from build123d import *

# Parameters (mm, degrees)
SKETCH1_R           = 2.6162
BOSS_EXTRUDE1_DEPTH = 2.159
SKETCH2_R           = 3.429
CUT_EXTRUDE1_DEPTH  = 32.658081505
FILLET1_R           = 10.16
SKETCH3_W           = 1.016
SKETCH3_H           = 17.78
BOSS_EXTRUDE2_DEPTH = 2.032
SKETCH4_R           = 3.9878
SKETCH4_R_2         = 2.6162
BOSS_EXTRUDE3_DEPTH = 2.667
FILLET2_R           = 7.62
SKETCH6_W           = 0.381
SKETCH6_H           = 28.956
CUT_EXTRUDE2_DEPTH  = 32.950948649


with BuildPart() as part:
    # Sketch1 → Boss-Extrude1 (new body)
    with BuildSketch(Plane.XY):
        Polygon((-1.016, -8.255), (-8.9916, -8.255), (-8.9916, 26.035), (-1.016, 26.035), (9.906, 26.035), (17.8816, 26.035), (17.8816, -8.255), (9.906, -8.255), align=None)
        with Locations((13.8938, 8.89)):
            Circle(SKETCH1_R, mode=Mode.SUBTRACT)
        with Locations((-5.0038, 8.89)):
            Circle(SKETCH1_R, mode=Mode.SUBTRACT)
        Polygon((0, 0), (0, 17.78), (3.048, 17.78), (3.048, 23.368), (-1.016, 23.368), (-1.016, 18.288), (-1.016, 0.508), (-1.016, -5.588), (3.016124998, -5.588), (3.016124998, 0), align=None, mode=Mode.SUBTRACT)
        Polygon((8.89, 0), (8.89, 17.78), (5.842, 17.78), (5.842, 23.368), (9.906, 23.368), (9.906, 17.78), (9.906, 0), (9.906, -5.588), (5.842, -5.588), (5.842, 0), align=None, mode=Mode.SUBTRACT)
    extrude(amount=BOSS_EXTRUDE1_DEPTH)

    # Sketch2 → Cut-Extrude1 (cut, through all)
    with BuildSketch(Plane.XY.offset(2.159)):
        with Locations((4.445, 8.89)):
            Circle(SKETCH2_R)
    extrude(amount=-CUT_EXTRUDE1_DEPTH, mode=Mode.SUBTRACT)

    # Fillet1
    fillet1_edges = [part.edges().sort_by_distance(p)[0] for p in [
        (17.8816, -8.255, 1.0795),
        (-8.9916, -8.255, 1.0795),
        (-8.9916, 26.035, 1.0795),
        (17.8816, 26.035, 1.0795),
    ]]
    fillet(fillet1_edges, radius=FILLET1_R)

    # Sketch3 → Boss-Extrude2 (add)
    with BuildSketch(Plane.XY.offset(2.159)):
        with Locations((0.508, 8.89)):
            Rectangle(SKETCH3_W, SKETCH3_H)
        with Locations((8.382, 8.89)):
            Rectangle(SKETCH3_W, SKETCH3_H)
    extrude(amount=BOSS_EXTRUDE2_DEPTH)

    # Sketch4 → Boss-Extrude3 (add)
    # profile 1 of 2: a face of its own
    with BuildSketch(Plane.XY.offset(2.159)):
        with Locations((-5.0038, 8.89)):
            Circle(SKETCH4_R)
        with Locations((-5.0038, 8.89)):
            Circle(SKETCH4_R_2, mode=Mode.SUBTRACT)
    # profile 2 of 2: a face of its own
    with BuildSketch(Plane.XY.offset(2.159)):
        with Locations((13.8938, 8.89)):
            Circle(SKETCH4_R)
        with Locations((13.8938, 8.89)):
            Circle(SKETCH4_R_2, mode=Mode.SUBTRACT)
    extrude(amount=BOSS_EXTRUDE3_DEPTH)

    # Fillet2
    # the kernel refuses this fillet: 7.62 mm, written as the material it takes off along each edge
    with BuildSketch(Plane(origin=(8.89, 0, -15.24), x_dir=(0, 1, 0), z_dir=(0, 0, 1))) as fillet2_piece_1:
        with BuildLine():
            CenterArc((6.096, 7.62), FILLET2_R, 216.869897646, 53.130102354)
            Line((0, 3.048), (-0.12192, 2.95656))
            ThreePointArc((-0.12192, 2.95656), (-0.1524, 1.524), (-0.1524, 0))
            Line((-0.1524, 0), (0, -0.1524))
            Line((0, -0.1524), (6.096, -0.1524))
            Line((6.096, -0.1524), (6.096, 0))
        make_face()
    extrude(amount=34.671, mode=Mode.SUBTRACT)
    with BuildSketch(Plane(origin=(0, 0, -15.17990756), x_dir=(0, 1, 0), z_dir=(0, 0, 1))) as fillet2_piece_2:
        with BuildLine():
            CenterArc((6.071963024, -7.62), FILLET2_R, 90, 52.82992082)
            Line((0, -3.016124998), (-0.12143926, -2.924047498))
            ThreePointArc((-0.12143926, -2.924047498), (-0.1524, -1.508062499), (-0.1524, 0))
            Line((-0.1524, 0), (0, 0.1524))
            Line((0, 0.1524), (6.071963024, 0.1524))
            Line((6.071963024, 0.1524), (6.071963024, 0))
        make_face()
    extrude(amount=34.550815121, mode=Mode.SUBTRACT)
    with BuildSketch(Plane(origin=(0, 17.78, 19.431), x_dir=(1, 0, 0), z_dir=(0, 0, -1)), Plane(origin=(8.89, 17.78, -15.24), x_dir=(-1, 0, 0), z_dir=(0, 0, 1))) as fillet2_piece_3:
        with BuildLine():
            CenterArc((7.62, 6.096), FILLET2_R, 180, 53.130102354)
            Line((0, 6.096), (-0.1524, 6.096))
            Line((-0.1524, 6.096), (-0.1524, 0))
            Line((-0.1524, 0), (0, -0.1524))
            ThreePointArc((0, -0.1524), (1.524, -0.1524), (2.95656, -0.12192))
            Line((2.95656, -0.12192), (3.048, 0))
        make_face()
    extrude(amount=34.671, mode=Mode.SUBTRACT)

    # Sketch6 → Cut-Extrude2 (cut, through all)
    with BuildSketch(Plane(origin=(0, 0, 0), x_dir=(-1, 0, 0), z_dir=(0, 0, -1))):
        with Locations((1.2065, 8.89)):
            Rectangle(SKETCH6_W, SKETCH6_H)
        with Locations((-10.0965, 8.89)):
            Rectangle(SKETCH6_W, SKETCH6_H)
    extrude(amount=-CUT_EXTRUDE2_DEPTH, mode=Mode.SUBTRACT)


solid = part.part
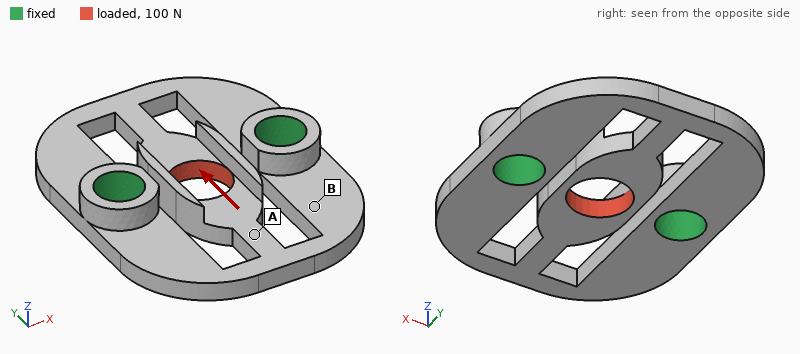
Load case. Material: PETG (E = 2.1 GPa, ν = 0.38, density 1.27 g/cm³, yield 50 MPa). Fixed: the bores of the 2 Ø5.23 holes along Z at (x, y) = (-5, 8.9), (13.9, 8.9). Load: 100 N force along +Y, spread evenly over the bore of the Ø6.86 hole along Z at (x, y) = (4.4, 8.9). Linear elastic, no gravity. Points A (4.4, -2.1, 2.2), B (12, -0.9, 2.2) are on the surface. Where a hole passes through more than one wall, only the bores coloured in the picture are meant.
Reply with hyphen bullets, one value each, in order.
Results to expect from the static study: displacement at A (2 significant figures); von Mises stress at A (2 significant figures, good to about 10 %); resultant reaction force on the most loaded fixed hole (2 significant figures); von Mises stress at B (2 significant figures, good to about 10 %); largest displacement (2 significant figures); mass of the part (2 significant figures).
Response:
- 0.18 mm
- 8.5 MPa
- 50 N
- 3.7 MPa
- 0.21 mm
- 1.8 g
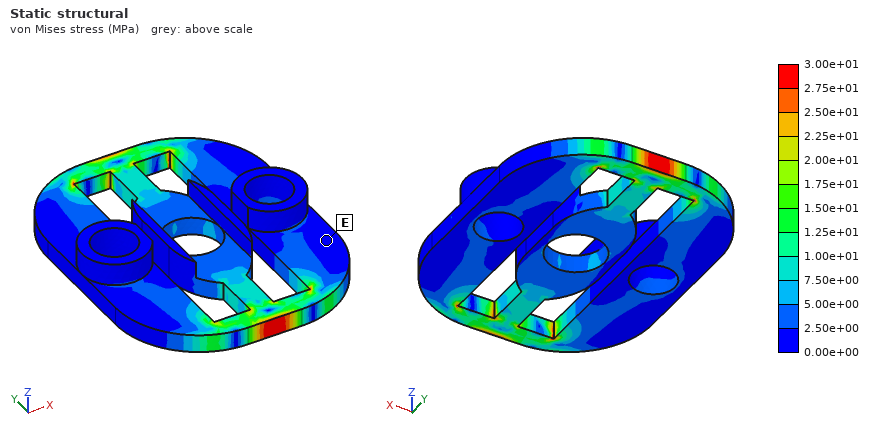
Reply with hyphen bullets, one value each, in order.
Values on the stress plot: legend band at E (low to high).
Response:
- 0.00e+00 to 2.50e+00 MPa
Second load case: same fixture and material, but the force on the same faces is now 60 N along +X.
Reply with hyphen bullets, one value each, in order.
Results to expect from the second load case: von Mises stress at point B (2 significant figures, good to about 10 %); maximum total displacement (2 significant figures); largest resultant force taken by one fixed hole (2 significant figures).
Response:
- 3.0 MPa
- 0.45 mm
- 30 N
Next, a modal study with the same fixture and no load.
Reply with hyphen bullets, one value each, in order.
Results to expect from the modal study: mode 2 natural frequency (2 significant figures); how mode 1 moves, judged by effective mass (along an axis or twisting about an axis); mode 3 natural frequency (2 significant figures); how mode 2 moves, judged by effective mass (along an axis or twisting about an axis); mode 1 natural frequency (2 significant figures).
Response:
- 1900 Hz
- along Z
- 2500 Hz
- twisting about X
- 1400 Hz
